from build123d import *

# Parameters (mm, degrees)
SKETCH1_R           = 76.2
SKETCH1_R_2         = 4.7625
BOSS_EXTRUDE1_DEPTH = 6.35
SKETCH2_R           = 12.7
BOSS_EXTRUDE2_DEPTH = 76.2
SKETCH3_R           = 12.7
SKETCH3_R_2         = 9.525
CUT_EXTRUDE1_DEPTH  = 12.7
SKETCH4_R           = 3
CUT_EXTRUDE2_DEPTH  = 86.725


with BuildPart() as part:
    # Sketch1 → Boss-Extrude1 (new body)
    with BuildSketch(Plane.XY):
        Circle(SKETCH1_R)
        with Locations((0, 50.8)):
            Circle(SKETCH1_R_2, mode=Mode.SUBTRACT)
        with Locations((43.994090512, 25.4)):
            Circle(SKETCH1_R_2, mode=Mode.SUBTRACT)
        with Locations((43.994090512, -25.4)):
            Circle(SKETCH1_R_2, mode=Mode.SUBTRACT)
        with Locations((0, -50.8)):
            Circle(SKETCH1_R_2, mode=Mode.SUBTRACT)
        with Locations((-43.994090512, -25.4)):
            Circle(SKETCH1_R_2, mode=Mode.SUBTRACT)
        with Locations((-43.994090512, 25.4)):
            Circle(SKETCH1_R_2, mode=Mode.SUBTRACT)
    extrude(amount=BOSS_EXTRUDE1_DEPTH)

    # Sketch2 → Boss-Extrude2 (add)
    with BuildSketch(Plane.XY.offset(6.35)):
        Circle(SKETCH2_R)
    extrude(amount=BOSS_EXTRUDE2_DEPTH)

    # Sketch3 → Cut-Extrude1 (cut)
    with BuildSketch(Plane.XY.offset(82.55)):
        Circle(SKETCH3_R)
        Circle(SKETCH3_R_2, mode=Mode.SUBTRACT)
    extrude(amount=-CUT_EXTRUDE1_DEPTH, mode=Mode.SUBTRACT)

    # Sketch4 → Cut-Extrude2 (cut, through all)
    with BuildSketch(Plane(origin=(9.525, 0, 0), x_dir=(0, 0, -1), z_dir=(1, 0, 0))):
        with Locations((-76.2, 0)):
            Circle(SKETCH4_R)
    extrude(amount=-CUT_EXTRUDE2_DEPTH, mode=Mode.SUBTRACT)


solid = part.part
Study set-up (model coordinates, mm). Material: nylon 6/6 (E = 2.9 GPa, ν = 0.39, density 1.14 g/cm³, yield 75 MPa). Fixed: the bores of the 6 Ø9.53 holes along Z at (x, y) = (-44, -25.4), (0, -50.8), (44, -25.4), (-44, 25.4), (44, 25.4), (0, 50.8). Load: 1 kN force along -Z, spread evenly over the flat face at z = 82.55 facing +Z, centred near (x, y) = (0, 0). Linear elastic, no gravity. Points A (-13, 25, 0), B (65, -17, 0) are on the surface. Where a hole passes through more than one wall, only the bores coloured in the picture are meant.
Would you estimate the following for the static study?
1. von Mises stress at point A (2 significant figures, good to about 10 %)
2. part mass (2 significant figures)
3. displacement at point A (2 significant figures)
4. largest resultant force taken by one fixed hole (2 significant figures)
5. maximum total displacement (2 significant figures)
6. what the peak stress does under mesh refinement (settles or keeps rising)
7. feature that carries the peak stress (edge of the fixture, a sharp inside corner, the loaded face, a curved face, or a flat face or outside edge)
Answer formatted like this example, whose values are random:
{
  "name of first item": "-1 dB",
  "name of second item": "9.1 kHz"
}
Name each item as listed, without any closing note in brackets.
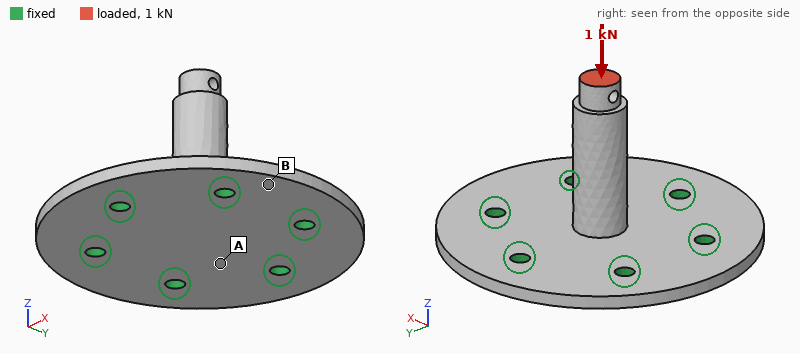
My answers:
{
  "von Mises stress at point A": "5.4 MPa",
  "part mass": "170 g",
  "displacement at point A": "0.22 mm",
  "largest resultant force taken by one fixed hole": "170 N",
  "maximum total displacement": "0.49 mm",
  "what the peak stress does under mesh refinement": "keeps rising",
  "feature that carries the peak stress": "edge of the fixture"
}
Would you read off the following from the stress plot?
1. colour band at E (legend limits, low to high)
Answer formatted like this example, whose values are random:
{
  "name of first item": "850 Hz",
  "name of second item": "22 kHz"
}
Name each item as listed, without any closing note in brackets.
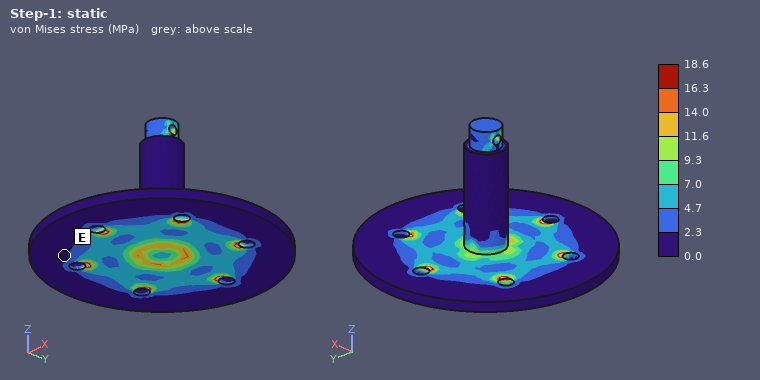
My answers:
{
  "colour band at E": "0.0 to 2.3 MPa"
}
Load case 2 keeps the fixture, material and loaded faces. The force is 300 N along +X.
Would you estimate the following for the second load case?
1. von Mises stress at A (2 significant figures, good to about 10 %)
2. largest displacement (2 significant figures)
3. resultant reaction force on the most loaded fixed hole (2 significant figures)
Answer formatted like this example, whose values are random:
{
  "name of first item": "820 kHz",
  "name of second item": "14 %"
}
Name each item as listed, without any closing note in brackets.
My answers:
{
  "von Mises stress at A": "6.2 MPa",
  "largest displacement": "2.4 mm",
  "resultant reaction force on the most loaded fixed hole": "200 N"
}
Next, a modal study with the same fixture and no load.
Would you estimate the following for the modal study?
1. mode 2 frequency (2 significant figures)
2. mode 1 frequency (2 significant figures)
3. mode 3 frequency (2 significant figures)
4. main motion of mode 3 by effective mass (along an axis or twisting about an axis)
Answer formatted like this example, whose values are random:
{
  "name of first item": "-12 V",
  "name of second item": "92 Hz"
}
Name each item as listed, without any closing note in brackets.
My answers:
{
  "mode 2 frequency": "550 Hz",
  "mode 1 frequency": "550 Hz",
  "mode 3 frequency": "1000 Hz",
  "main motion of mode 3 by effective mass": "along Z"
}
